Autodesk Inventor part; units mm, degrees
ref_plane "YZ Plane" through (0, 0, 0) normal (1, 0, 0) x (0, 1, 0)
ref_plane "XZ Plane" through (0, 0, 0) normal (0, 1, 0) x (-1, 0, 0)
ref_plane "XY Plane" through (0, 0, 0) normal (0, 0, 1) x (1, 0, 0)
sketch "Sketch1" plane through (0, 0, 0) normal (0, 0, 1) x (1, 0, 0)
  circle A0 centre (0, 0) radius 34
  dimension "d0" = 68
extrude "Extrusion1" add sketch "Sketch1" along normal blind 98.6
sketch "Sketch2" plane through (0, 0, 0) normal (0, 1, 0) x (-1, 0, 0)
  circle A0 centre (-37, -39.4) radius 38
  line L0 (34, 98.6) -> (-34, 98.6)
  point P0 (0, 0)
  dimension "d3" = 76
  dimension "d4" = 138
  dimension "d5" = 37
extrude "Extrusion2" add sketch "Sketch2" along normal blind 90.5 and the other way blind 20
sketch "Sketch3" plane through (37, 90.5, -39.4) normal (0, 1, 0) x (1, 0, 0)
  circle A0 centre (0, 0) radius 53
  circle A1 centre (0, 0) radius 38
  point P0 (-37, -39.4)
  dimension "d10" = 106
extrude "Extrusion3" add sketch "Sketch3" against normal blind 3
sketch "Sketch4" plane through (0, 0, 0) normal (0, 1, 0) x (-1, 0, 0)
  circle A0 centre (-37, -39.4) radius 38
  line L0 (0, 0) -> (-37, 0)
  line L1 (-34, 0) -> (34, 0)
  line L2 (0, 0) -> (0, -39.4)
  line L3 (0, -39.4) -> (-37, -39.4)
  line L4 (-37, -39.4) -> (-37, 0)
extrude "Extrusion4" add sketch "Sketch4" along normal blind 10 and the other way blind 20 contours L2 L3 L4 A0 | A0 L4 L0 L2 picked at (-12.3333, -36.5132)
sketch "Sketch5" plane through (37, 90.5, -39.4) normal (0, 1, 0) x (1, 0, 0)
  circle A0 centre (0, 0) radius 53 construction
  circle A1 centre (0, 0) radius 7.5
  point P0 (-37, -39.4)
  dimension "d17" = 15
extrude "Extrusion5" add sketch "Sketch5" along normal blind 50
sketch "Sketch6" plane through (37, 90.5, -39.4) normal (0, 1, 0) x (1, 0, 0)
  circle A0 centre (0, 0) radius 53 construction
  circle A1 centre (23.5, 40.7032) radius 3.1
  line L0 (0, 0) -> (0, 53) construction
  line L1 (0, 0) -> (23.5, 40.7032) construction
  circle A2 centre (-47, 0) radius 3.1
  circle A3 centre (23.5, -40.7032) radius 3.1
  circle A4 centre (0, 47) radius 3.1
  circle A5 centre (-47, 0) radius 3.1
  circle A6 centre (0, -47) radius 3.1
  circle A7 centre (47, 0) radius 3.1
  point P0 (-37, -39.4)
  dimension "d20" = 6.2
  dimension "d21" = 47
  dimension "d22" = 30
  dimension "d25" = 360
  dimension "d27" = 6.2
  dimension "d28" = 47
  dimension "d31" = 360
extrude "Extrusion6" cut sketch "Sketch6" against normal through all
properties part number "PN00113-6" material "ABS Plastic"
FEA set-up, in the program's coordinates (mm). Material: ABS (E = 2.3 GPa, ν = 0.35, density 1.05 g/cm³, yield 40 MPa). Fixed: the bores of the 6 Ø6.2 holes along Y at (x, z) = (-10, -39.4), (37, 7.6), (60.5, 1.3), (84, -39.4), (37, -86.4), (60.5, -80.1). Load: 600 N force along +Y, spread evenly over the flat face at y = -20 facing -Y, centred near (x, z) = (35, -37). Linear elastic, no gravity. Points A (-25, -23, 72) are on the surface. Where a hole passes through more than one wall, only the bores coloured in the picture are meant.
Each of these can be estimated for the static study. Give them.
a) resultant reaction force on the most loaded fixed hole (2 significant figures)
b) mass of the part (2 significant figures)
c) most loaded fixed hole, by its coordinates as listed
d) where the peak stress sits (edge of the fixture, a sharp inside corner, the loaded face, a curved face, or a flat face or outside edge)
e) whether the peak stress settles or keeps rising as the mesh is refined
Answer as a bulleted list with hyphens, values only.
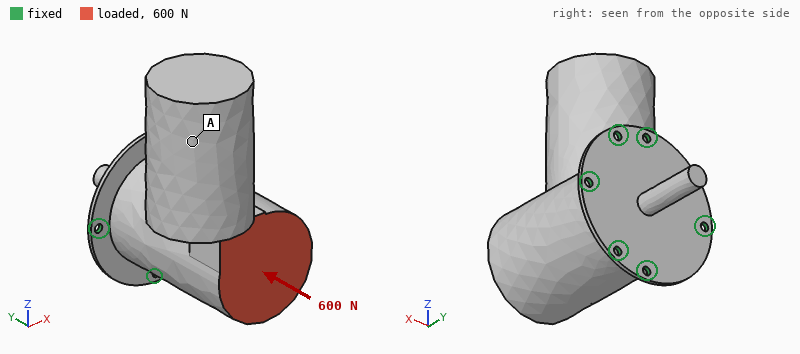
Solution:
- 180 N
- 930 g
- (-10, -39.4)
- edge of the fixture
- keeps rising
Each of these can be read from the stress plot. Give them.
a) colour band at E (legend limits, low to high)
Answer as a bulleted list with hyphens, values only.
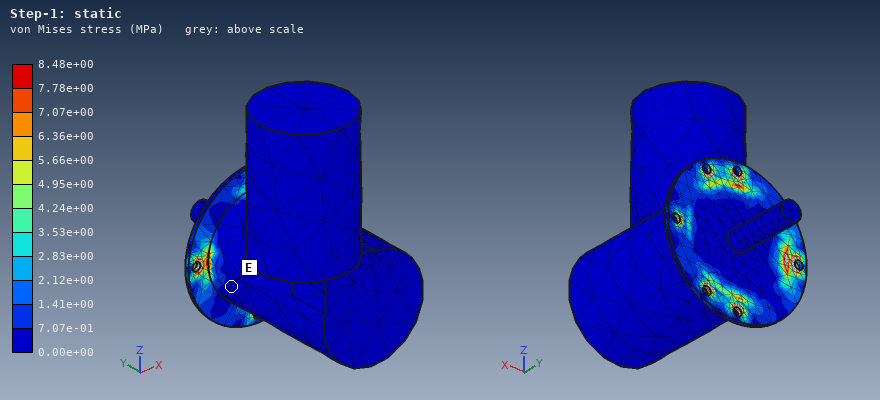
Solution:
- 0.00e+00 to 7.07e-01 MPa
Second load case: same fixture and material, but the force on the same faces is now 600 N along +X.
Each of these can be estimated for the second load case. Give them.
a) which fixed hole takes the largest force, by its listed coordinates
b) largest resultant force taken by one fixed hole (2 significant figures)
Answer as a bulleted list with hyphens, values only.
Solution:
- (-10, -39.4)
- 830 N
